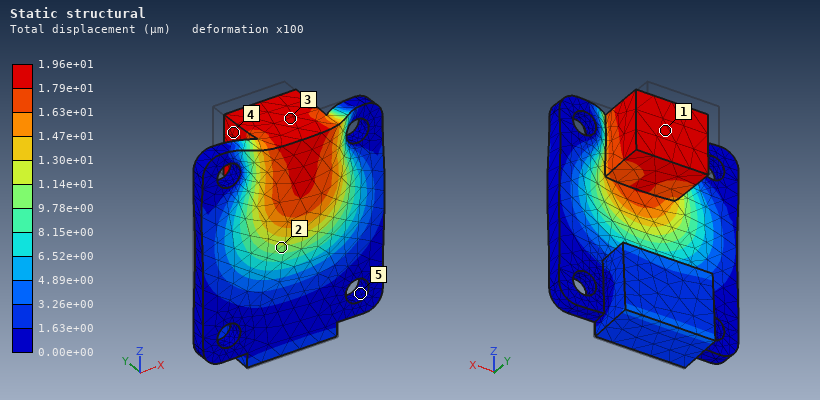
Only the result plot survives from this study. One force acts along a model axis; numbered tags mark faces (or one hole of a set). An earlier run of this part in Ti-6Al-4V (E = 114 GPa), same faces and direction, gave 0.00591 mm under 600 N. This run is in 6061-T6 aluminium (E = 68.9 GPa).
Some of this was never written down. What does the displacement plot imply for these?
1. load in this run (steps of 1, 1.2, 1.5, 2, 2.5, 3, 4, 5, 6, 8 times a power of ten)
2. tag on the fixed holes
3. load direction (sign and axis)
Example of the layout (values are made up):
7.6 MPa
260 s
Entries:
1.2 kN
5
-Y
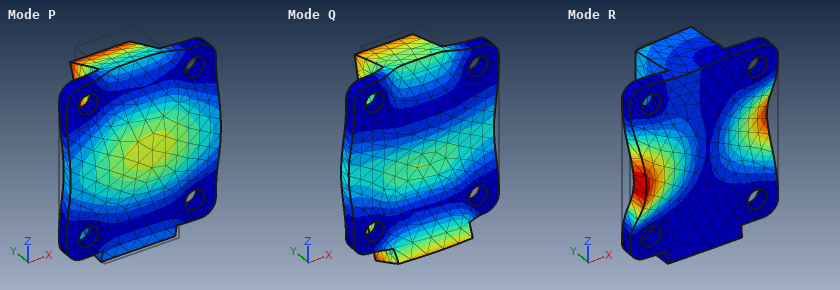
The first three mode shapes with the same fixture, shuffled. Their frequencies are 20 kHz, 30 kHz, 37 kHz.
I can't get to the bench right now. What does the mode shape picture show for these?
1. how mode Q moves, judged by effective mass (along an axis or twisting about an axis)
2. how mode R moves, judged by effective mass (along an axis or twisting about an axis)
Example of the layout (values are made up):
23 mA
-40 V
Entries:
along Z
twisting about Z
